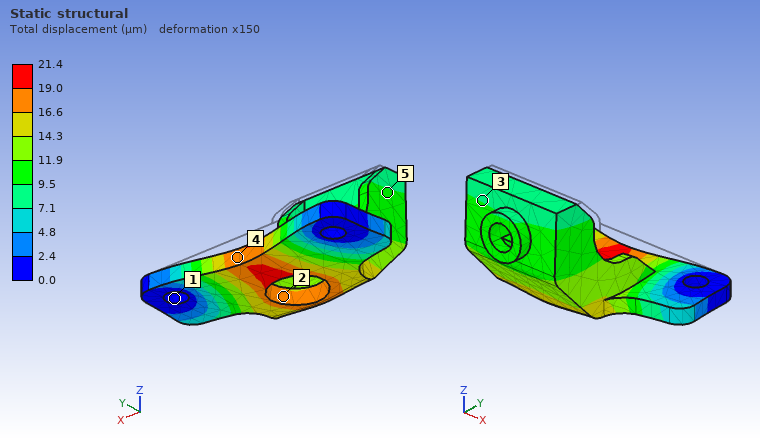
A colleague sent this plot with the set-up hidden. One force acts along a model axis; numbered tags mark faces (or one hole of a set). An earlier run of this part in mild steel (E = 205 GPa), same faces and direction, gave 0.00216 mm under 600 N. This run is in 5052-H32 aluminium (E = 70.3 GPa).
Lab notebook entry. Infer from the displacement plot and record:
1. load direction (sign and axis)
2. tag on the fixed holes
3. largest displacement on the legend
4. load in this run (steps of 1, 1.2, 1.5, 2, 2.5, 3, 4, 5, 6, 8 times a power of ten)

-Y
1
21.4 µm
2 kN
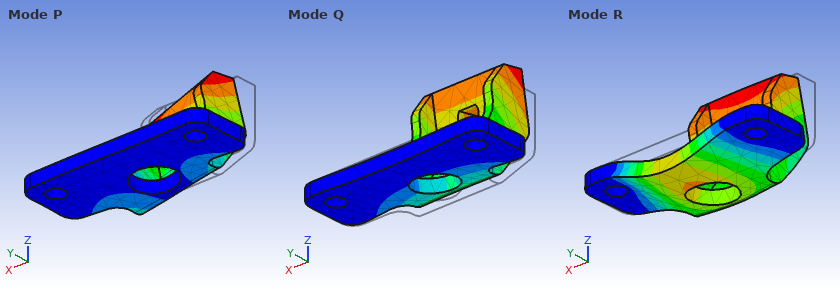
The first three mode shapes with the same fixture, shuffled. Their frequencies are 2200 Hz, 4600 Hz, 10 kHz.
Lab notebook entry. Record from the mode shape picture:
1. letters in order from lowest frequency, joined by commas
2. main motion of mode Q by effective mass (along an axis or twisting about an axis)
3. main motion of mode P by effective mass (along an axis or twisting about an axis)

Q, P, R
along Z
along X
